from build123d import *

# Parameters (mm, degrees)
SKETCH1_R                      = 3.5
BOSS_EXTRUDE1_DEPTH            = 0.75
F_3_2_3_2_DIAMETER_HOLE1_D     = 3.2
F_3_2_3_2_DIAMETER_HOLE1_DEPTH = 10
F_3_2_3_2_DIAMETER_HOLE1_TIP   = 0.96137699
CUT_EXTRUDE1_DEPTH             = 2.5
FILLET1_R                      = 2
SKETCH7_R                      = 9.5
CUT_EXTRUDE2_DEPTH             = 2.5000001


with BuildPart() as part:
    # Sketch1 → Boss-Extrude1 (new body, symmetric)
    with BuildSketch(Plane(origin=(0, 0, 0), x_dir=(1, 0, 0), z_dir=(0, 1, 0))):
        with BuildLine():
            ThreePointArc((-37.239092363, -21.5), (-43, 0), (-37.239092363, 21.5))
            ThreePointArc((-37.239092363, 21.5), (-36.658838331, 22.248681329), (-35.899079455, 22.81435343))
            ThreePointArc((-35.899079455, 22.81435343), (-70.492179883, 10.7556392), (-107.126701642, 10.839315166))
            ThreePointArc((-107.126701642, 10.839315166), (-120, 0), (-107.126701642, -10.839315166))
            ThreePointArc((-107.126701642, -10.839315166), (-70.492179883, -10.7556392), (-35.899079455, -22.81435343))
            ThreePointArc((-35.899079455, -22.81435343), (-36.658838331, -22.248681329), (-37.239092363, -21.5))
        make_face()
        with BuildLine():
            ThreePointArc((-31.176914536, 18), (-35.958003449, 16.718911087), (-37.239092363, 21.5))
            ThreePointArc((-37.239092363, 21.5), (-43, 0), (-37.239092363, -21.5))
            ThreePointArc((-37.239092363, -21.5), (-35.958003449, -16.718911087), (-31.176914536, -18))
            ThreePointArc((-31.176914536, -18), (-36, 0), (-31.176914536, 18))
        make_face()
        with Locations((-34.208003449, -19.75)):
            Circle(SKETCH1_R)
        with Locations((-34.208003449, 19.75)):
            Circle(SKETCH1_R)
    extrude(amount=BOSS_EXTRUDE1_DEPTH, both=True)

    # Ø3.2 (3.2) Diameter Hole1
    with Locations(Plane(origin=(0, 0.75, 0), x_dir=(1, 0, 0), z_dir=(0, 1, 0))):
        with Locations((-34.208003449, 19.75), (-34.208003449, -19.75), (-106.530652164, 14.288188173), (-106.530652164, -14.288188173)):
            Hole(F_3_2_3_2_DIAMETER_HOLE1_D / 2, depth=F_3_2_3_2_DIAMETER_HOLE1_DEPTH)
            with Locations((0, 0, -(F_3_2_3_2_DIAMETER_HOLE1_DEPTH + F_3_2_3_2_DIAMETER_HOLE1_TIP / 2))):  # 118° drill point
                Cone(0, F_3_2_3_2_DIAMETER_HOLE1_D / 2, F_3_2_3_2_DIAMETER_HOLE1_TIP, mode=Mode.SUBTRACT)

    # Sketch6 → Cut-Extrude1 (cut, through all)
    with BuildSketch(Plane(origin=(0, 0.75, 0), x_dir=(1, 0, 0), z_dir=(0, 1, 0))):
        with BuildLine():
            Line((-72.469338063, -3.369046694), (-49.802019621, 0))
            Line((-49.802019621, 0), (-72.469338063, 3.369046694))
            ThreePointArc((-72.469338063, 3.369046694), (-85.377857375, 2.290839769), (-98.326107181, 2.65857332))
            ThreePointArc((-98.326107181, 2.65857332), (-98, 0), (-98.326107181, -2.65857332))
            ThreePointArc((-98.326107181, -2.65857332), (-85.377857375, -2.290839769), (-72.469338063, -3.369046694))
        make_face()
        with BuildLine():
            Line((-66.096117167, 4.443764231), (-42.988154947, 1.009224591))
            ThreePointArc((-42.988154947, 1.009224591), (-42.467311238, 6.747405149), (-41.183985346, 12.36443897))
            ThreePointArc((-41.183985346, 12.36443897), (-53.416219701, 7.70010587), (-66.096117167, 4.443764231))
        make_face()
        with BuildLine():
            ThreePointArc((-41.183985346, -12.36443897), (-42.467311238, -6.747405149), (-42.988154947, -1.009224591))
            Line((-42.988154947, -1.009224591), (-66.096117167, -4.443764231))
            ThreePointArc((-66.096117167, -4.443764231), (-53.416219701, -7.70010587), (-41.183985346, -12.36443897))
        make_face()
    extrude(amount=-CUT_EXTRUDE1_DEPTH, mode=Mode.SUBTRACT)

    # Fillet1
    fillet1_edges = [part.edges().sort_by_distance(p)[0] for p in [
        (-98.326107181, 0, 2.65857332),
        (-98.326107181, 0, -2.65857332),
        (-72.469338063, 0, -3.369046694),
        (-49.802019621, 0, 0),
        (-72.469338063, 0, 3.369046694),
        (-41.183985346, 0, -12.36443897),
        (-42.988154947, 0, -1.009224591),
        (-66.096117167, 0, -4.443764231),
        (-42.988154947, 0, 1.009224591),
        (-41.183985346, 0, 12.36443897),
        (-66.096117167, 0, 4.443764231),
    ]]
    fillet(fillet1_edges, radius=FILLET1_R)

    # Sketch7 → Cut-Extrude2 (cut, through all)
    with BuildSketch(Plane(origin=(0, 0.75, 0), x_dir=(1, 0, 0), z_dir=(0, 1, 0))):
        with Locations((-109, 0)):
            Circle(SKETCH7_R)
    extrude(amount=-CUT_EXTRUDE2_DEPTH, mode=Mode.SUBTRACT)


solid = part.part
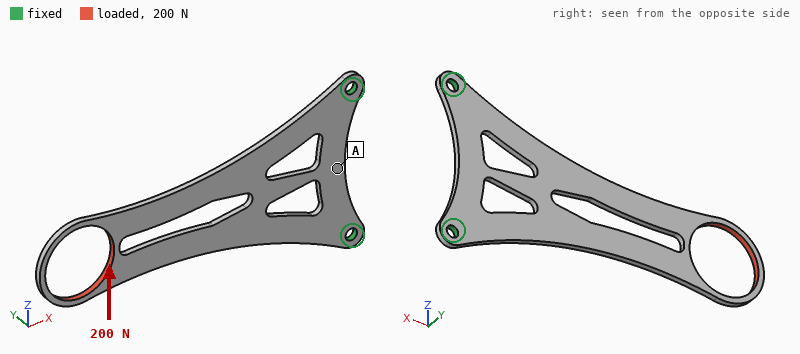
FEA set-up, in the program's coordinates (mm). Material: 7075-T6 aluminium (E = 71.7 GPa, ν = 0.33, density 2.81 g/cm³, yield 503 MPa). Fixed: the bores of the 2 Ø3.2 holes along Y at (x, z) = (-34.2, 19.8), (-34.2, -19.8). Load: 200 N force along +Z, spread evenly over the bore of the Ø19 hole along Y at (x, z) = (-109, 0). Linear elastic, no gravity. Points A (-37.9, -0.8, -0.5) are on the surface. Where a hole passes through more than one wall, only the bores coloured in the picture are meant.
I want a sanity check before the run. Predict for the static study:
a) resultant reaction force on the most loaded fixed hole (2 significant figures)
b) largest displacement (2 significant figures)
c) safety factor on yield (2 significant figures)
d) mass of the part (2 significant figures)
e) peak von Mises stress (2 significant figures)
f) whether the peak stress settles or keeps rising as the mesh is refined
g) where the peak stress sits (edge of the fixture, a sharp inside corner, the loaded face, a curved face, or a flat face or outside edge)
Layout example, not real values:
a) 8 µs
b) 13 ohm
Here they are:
a) 410 N
b) 0.83 mm
c) 0.76
d) 6.1 g
e) 660 MPa
f) settles
g) a curved face
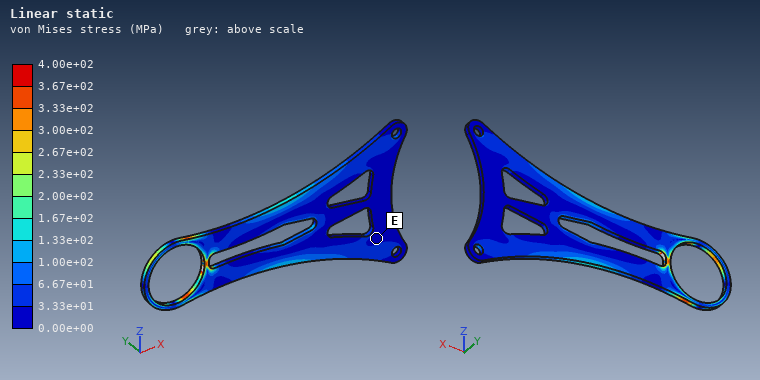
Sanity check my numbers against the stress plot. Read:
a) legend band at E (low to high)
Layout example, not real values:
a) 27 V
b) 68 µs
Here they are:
a) 0.00e+00 to 3.33e+01 MPa
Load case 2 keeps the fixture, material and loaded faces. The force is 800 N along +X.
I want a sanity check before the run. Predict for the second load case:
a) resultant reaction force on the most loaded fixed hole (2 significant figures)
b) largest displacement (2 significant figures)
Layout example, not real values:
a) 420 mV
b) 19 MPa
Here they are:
a) 470 N
b) 0.29 mm
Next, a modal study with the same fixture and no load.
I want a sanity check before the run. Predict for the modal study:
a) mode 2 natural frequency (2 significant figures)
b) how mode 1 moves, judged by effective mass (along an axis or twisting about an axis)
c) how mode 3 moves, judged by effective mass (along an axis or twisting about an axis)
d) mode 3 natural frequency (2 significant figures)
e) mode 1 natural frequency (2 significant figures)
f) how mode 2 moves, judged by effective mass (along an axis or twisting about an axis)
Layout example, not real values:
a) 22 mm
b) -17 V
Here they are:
a) 1200 Hz
b) along Y
c) twisting about X
d) 1600 Hz
e) 250 Hz
f) along Y
